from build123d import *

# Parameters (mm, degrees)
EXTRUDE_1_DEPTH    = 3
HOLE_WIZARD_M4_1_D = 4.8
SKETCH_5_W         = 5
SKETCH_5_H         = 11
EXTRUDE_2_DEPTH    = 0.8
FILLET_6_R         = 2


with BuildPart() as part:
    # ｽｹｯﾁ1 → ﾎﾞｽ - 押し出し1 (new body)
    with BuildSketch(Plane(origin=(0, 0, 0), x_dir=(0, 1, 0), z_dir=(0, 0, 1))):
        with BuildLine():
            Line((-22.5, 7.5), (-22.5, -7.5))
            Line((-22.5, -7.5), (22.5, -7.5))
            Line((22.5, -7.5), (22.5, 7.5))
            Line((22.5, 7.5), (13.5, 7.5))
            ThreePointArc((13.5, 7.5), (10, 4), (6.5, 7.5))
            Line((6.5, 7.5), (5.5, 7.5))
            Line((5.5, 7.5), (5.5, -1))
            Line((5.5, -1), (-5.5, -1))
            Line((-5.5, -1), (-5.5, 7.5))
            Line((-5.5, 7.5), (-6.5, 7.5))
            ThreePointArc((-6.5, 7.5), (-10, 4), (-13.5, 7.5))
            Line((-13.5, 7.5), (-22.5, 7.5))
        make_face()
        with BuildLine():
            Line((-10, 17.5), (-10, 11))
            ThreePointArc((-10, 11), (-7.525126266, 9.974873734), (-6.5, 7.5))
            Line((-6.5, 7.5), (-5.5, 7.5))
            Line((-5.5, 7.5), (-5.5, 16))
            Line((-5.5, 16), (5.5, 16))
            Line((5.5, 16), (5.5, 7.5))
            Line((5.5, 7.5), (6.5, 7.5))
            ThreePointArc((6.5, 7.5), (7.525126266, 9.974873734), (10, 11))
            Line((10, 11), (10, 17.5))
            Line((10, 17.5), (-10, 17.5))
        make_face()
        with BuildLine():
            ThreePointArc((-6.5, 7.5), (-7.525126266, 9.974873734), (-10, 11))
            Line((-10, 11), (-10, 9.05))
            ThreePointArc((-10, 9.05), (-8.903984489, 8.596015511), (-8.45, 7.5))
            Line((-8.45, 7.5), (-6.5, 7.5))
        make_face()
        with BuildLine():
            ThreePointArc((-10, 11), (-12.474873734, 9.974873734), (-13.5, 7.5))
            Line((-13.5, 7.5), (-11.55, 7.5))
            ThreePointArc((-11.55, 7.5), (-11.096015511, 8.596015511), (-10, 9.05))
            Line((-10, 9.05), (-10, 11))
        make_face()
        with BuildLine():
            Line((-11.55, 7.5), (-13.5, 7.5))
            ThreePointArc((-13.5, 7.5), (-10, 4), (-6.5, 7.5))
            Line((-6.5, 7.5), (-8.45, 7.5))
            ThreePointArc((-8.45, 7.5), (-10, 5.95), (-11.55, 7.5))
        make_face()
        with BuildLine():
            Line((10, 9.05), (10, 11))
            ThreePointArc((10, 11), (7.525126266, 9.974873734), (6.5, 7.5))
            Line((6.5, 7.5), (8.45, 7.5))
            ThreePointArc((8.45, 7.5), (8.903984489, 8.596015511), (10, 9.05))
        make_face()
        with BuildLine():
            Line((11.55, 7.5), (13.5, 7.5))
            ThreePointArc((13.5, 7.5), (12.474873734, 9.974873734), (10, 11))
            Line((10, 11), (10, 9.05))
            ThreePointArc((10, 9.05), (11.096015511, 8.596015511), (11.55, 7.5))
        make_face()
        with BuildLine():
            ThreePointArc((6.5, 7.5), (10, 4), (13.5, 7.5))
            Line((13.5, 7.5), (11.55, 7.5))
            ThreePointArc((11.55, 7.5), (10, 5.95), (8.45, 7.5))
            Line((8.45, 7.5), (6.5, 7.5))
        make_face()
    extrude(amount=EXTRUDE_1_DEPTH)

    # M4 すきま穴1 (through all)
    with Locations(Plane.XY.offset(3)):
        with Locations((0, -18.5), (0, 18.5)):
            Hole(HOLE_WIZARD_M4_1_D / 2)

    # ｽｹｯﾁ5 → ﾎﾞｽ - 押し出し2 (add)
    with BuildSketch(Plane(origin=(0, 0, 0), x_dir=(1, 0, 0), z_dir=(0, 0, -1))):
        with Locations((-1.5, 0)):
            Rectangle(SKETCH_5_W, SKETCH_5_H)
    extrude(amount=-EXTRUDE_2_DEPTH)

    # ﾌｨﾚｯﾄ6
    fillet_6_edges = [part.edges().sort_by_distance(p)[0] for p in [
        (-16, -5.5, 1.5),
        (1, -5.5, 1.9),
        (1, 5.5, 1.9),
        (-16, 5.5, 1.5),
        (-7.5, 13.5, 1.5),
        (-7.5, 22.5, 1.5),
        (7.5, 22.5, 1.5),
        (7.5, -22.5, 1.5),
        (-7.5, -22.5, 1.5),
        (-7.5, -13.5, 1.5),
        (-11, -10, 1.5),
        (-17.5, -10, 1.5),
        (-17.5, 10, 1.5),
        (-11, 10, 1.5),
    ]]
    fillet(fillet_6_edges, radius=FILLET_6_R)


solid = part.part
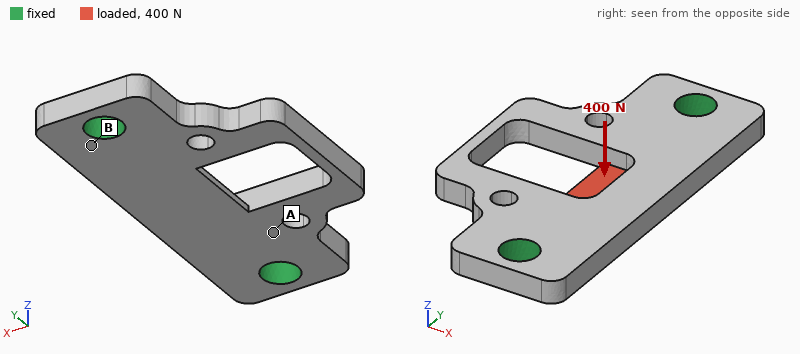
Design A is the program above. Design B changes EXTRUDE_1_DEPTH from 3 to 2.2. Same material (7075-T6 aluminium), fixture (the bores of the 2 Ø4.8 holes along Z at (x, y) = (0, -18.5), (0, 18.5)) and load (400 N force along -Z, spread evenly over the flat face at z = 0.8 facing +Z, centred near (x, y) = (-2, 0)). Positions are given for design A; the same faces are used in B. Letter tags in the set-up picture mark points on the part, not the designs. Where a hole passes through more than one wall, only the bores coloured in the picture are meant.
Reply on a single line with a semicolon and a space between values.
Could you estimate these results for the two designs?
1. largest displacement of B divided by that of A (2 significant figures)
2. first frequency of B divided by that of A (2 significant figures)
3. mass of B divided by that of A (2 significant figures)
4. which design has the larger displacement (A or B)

1.6; 0.76; 0.74; B
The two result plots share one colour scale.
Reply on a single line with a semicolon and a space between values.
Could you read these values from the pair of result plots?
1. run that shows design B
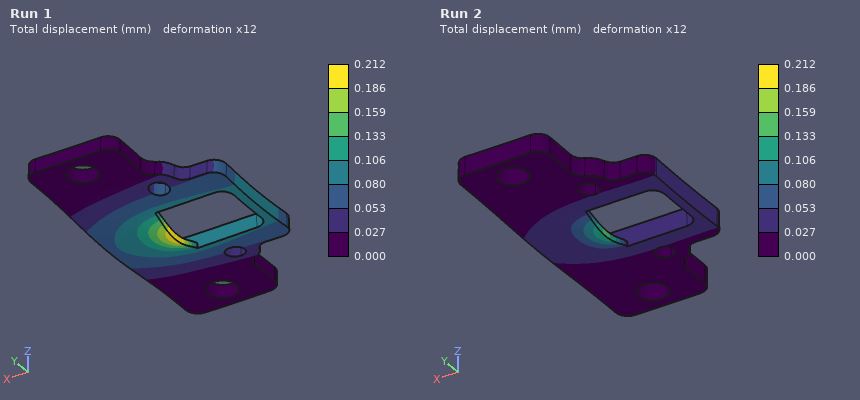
Run 1
